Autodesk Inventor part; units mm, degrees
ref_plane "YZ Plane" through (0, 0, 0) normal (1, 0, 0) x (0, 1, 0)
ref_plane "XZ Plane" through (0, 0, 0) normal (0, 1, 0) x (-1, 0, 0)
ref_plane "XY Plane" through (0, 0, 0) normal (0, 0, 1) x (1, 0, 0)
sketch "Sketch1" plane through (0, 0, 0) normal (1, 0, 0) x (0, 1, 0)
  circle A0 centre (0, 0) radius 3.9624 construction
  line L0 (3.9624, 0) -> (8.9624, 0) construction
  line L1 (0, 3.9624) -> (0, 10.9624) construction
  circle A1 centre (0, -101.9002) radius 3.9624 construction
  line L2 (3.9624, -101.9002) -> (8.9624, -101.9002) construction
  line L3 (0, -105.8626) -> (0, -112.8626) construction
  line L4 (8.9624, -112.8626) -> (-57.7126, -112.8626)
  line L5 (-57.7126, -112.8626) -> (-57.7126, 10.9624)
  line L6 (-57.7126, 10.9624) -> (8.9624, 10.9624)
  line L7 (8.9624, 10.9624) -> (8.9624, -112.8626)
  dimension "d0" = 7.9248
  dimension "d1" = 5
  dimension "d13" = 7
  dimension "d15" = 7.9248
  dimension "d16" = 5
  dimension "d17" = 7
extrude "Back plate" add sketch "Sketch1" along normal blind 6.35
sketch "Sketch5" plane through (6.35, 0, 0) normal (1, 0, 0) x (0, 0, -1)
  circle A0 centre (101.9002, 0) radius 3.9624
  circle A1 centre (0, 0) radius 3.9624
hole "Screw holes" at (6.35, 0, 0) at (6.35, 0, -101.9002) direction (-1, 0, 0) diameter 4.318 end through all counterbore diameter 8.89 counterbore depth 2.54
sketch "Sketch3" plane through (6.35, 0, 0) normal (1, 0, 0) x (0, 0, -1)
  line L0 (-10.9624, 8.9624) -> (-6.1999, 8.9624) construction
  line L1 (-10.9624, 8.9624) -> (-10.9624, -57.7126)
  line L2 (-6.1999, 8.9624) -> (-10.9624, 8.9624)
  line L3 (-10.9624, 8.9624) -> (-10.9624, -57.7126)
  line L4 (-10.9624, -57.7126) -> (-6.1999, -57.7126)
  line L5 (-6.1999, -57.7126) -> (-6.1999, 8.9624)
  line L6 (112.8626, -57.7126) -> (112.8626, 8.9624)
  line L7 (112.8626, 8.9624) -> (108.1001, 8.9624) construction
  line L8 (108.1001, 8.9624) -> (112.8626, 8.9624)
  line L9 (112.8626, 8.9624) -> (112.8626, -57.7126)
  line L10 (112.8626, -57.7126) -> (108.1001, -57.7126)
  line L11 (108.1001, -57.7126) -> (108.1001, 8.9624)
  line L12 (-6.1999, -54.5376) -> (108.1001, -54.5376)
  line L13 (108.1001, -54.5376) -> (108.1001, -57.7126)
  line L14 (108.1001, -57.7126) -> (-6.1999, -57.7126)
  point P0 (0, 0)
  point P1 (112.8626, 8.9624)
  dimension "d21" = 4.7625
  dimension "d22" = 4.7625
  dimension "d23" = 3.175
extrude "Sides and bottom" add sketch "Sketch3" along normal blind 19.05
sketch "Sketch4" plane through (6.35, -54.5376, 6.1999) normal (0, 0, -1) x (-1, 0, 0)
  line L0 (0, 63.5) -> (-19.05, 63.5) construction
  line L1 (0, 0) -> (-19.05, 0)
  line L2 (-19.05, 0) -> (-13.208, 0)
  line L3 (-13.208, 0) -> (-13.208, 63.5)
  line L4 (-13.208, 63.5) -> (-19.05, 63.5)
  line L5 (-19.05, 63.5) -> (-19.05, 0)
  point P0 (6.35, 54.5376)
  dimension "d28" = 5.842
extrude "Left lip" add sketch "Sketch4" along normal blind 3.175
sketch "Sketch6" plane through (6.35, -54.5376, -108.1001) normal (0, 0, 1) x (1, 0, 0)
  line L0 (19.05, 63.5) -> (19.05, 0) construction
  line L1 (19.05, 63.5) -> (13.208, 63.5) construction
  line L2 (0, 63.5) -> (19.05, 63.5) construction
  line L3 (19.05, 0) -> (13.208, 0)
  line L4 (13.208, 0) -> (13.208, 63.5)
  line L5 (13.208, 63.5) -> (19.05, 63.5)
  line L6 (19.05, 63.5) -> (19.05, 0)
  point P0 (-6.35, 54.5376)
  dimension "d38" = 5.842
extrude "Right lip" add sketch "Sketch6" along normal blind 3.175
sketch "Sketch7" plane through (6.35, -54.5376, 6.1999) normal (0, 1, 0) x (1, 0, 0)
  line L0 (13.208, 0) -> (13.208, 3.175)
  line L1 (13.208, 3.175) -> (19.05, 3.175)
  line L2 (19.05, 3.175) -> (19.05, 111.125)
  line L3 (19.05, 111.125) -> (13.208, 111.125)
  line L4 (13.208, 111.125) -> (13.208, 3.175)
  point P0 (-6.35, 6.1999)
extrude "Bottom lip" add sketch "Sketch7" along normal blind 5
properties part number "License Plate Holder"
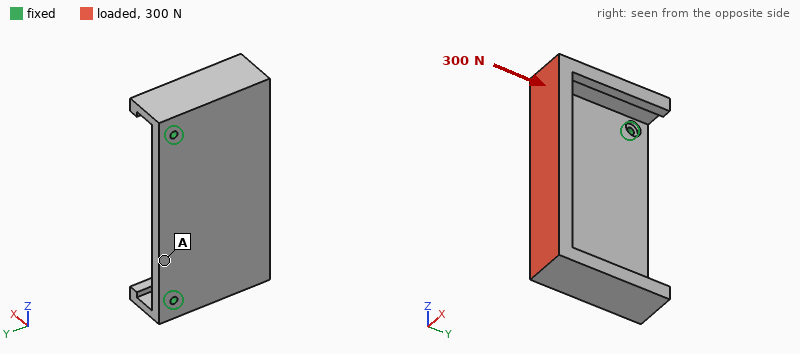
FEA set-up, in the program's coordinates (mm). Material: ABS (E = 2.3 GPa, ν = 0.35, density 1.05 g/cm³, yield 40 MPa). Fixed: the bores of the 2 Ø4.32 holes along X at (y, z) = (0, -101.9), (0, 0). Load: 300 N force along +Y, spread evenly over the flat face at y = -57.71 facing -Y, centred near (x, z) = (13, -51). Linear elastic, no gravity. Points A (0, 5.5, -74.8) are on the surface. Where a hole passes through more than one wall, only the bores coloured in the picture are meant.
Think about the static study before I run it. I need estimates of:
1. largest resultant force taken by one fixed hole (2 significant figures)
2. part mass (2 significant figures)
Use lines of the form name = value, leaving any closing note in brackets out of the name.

largest resultant force taken by one fixed hole = 150 N
part mass = 80 g
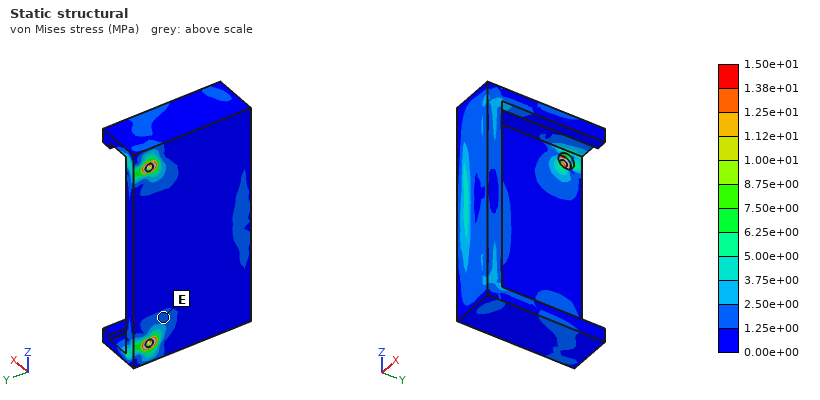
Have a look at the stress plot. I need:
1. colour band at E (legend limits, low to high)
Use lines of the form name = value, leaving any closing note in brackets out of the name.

colour band at E = 1.25e+00 to 2.50e+00 MPa
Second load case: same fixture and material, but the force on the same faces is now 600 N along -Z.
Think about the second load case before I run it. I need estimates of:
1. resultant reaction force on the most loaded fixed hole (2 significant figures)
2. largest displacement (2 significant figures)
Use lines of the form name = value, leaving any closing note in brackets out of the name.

resultant reaction force on the most loaded fixed hole = 450 N
largest displacement = 0.94 mm
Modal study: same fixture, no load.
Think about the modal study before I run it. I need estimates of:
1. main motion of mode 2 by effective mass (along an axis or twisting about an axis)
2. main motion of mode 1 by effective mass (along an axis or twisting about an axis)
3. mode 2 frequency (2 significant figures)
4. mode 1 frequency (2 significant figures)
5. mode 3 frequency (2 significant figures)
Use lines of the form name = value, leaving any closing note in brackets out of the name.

main motion of mode 2 by effective mass = twisting about Y
main motion of mode 1 by effective mass = along X
mode 2 frequency = 420 Hz
mode 1 frequency = 210 Hz
mode 3 frequency = 830 Hz
